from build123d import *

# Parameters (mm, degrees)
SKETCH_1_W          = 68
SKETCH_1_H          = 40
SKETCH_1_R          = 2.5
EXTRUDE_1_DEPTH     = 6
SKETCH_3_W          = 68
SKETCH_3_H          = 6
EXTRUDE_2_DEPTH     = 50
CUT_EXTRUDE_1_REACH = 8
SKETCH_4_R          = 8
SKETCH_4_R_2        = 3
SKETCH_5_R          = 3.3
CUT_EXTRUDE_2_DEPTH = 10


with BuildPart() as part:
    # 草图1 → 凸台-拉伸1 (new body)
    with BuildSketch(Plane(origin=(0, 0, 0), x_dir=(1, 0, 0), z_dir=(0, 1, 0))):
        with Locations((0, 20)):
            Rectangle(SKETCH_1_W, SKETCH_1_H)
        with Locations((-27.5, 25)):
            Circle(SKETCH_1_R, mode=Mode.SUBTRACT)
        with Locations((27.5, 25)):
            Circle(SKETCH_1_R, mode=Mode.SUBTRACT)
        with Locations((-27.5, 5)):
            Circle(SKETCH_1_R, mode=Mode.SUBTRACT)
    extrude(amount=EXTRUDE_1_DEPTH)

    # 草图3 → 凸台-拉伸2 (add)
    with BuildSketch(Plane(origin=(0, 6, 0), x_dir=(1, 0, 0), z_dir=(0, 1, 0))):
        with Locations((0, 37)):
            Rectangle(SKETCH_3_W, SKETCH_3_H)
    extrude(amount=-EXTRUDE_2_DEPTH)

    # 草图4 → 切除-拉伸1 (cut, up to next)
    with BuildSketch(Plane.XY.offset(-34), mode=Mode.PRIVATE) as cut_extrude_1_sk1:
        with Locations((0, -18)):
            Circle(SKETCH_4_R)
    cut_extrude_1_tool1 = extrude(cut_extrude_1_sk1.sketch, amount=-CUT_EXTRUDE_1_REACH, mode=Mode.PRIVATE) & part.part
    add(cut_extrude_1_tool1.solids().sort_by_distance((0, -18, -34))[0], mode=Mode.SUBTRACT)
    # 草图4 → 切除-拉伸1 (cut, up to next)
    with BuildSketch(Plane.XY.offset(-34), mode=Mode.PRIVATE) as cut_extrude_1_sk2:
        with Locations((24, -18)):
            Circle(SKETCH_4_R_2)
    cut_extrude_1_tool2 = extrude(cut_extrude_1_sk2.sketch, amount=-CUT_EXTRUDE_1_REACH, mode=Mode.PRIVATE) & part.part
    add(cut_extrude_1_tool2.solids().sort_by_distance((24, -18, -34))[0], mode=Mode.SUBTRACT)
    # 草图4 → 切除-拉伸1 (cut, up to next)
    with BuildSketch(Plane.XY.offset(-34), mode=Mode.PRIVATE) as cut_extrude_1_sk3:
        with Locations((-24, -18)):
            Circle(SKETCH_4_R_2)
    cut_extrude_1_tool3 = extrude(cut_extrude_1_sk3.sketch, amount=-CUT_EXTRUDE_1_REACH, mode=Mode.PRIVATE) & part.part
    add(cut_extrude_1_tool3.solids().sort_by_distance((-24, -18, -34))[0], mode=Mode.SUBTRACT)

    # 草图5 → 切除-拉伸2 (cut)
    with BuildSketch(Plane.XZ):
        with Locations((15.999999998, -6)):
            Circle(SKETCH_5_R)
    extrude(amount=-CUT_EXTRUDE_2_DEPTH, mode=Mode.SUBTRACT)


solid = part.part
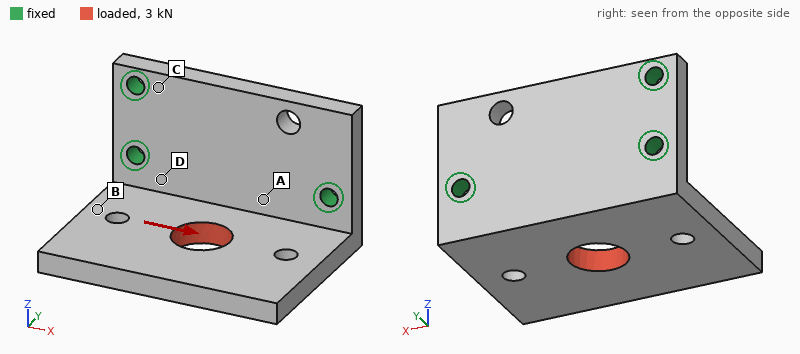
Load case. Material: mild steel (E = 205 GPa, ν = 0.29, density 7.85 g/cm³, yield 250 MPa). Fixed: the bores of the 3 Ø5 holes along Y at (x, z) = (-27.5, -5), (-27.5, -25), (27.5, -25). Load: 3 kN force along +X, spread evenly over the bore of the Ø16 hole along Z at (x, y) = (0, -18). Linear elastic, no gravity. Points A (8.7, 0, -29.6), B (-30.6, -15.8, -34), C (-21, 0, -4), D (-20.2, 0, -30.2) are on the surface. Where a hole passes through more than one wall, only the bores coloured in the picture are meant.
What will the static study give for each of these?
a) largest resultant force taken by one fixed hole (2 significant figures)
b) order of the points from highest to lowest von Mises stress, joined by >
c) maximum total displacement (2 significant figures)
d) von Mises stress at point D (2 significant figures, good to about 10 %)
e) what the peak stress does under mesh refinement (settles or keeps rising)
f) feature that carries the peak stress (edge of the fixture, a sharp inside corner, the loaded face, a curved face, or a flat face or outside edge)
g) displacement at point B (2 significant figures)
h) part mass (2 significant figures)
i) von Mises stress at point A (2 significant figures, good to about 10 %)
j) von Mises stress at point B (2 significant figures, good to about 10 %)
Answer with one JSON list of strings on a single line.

["1.9 kN", "D > A > B > C", "24 µm", "39 MPa", "keeps rising", "edge of the fixture", "13 µm", "250 g", "25 MPa", "17 MPa"]
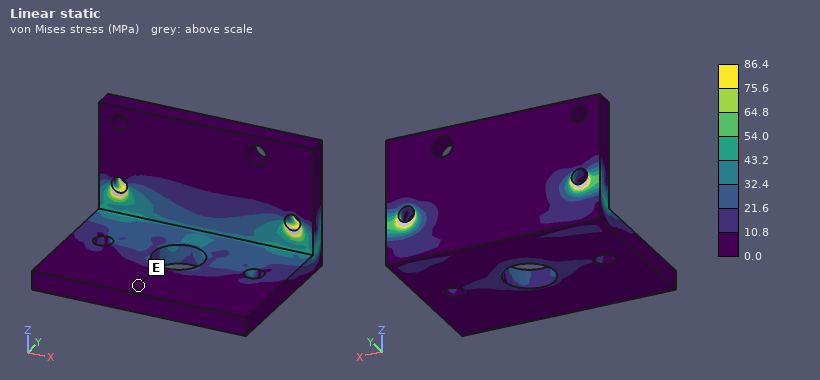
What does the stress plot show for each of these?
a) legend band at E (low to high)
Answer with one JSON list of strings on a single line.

["0.0 to 10.8 MPa"]
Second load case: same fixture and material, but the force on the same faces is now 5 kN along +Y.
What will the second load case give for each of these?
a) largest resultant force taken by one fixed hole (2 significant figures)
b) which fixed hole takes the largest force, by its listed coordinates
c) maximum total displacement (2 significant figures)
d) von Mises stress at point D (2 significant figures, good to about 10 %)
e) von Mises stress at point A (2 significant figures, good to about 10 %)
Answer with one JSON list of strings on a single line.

["3.0 kN", "(-27.5, -25)", "95 µm", "75 MPa", "37 MPa"]
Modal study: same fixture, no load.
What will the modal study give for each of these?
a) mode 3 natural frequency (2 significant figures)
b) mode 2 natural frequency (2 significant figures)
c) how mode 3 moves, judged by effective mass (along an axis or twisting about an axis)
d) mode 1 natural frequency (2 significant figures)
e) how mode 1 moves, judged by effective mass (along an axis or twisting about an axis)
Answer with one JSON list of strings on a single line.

["6100 Hz", "3400 Hz", "along X", "1500 Hz", "along Z"]
